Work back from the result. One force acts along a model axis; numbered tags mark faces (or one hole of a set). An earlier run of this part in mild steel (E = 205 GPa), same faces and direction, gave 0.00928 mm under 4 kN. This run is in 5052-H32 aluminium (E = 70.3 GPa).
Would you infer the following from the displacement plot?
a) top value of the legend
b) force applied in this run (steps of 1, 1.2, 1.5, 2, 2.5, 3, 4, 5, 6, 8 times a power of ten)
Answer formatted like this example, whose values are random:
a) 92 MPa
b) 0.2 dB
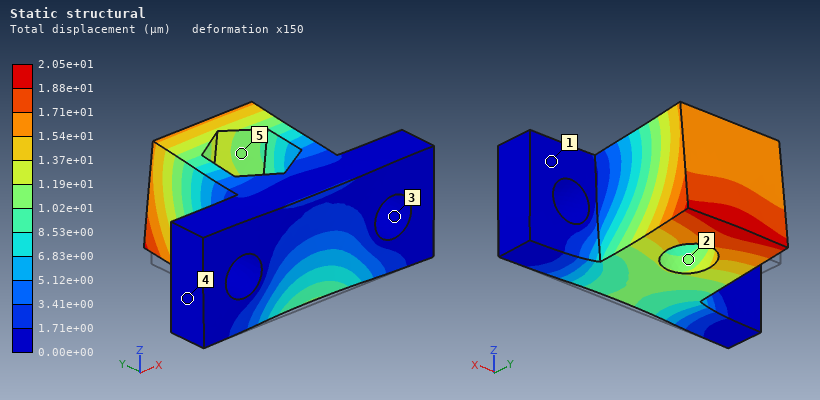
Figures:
a) 2.05e+01 µm
b) 3 kN
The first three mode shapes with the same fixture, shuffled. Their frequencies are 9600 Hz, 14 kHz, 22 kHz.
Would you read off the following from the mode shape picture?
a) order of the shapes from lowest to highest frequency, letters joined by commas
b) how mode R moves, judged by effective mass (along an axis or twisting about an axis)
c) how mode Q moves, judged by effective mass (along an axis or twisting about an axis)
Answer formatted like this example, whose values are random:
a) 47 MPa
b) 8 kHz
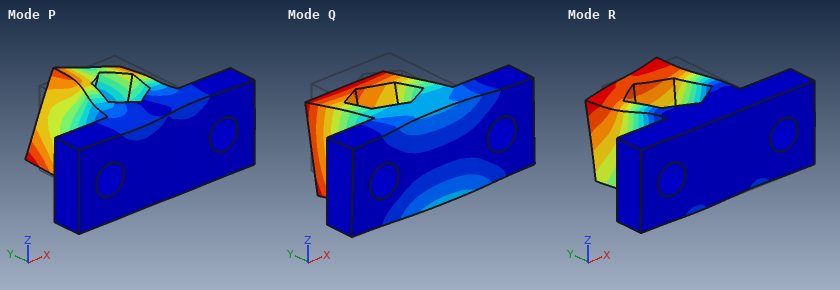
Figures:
a) Q, R, P
b) along X
c) along Z
